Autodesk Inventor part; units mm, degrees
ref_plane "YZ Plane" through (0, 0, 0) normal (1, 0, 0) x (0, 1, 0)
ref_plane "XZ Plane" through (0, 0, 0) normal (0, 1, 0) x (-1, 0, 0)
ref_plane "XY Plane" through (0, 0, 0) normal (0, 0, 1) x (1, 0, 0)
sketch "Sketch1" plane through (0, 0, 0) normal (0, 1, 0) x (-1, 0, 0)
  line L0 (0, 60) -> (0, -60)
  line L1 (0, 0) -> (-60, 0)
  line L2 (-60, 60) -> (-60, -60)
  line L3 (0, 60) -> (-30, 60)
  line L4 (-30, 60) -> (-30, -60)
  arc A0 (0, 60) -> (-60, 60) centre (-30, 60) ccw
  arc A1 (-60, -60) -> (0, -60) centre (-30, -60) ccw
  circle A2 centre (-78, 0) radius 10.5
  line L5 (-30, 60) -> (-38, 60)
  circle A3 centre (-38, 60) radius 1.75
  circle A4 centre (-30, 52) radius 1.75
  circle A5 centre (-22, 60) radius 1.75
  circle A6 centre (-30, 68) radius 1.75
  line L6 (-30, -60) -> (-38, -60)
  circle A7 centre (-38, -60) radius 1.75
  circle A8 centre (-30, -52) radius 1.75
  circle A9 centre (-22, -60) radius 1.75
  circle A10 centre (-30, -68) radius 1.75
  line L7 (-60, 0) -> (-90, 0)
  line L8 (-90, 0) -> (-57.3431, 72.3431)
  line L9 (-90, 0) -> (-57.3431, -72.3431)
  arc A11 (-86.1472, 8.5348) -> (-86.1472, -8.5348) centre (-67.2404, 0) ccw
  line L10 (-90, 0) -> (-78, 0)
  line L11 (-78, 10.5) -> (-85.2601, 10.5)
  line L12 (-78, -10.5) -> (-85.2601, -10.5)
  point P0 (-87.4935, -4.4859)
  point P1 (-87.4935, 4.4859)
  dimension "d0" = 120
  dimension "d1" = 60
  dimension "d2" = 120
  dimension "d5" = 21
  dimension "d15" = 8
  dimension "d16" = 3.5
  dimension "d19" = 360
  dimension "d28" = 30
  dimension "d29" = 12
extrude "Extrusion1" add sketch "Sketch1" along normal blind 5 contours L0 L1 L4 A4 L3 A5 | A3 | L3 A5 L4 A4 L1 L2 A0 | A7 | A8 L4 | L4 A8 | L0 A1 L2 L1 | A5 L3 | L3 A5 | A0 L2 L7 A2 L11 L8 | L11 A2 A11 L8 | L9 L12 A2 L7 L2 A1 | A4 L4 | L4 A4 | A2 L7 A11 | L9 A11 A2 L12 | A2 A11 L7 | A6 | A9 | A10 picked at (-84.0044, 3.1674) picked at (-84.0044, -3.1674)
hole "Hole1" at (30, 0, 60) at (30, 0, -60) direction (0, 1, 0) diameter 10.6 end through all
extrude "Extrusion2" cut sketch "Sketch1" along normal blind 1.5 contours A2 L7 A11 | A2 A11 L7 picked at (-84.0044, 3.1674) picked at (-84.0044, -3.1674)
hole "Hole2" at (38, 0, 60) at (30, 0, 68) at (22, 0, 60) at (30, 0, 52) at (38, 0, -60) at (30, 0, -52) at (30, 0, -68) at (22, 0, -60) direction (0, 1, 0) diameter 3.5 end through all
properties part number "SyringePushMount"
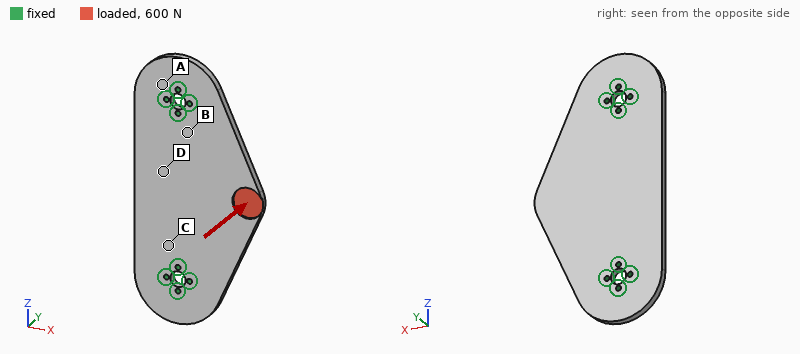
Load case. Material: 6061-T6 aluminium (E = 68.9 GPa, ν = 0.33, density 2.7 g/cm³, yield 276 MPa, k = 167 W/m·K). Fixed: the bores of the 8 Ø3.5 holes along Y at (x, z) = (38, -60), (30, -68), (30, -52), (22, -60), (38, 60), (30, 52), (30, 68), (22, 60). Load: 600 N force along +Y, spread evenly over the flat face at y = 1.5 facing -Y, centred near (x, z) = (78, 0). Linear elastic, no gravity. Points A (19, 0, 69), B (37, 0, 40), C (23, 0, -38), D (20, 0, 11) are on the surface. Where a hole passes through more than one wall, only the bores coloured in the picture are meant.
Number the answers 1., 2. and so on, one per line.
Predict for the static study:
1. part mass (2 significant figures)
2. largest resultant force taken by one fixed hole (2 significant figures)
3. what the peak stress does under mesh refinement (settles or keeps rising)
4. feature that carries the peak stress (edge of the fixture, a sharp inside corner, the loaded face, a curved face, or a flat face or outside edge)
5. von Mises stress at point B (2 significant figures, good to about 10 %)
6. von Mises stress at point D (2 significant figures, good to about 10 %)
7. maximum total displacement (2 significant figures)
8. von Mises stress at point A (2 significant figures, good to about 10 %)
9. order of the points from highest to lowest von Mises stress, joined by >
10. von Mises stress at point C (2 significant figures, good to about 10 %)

1. 160 g
2. 470 N
3. keeps rising
4. edge of the fixture
5. 43 MPa
6. 16 MPa
7. 0.67 mm
8. 8.7 MPa
9. B > C > D > A
10. 32 MPa
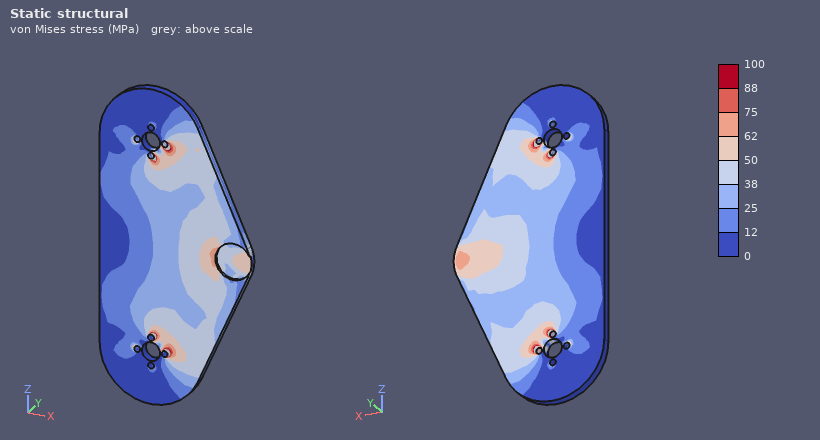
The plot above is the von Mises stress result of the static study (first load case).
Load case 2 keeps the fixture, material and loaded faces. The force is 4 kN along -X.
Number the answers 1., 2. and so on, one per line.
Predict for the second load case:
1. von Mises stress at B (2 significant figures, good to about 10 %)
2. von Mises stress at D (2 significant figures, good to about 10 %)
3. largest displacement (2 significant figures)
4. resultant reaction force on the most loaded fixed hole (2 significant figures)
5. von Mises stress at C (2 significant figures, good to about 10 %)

1. 20 MPa
2. 6.6 MPa
3. 0.14 mm
4. 1.5 kN
5. 14 MPa
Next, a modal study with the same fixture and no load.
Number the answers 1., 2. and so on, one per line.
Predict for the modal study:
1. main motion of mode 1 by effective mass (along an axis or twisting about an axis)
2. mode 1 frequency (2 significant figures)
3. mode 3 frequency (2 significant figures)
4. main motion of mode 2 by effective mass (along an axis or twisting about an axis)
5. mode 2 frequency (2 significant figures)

1. along Y
2. 1300 Hz
3. 3500 Hz
4. along Y
5. 2100 Hz
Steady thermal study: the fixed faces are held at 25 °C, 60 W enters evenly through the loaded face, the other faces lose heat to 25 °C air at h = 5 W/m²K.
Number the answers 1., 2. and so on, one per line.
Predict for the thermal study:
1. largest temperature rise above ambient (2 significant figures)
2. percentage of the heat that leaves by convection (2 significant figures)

1. 72 K
2. 3.2 %
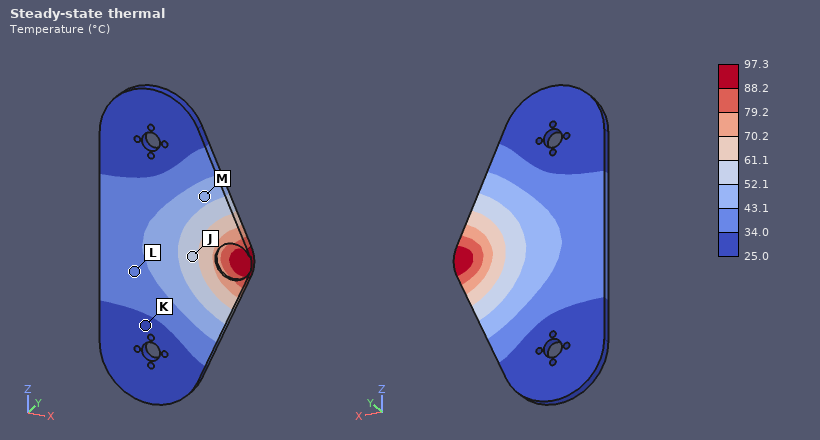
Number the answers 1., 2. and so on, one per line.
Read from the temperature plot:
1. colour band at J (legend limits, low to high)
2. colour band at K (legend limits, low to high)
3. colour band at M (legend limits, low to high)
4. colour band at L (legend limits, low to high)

1. 52.1 to 61.1 °C
2. 25.0 to 34.0 °C
3. 43.1 to 52.1 °C
4. 34.0 to 43.1 °C
